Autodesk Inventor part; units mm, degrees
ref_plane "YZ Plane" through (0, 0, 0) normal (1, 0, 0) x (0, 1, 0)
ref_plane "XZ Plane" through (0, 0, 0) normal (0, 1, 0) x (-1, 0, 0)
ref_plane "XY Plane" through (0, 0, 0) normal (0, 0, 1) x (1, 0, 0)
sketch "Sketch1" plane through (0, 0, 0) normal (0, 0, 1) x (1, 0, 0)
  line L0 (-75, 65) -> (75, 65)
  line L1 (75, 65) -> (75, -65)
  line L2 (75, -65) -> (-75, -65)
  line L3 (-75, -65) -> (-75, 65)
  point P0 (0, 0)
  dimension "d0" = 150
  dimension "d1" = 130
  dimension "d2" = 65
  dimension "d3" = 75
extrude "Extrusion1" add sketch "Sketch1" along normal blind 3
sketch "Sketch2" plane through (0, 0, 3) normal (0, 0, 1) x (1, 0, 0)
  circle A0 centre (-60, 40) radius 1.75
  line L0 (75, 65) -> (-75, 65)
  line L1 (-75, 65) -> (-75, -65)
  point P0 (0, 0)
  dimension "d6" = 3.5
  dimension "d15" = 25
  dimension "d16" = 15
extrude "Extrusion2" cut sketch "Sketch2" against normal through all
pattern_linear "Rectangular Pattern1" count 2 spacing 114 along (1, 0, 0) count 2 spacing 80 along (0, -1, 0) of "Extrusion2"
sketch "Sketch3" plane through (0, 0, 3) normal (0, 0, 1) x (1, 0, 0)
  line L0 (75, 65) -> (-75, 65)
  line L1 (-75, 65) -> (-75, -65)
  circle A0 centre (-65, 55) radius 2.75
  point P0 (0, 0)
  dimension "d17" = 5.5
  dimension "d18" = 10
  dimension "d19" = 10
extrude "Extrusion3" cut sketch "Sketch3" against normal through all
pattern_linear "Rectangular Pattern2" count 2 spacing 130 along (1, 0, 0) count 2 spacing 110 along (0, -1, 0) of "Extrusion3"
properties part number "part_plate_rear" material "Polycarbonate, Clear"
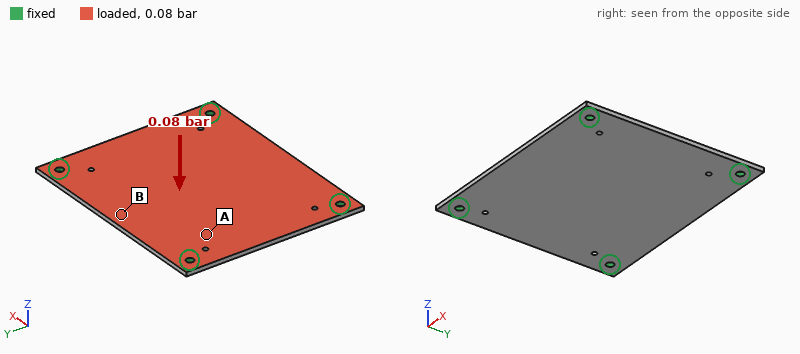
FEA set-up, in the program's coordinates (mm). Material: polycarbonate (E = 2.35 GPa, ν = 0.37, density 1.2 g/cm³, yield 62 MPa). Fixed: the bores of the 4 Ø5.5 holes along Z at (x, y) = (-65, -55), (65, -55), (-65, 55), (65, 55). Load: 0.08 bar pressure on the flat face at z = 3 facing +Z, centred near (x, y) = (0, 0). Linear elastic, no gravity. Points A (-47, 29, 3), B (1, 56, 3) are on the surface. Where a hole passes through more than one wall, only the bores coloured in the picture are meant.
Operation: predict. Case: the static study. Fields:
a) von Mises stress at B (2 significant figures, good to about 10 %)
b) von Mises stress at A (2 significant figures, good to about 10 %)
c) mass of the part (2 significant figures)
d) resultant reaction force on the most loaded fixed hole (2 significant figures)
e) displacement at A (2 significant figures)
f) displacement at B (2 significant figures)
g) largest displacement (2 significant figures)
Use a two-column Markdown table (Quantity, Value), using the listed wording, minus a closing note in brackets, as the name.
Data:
| Quantity | Value |
|---|---|
| von Mises stress at B | 4.9 MPa |
| von Mises stress at A | 1.7 MPa |
| mass of the part | 70 g |
| resultant reaction force on the most loaded fixed hole | 39 N |
| displacement at A | 0.93 mm |
| displacement at B | 1.5 mm |
| largest displacement | 2.2 mm |
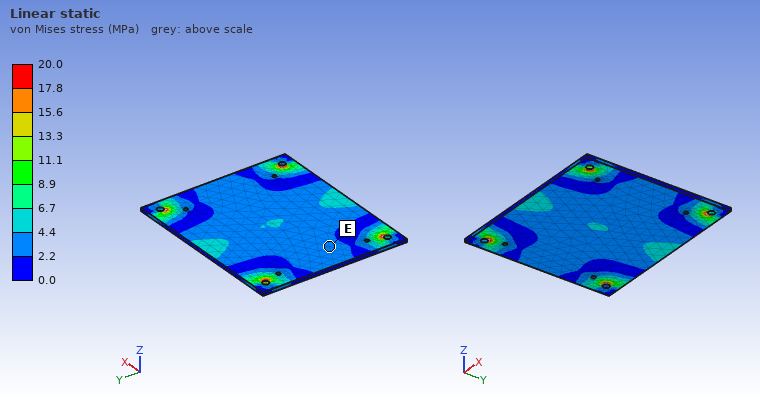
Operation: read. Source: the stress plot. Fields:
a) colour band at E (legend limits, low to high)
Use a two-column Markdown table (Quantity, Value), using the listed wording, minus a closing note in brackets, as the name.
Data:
| Quantity | Value |
|---|---|
| colour band at E | 2.2 to 4.4 MPa |
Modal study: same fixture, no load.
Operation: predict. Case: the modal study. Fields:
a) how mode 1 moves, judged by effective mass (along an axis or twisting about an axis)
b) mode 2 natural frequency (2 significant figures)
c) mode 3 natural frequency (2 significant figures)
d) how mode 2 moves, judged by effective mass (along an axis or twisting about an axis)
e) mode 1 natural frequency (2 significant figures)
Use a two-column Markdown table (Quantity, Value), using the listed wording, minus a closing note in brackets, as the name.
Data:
| Quantity | Value |
|---|---|
| how mode 1 moves, judged by effective mass | along Z |
| mode 2 natural frequency | 310 Hz |
| mode 3 natural frequency | 380 Hz |
| how mode 2 moves, judged by effective mass | twisting about X |
| mode 1 natural frequency | 190 Hz |
